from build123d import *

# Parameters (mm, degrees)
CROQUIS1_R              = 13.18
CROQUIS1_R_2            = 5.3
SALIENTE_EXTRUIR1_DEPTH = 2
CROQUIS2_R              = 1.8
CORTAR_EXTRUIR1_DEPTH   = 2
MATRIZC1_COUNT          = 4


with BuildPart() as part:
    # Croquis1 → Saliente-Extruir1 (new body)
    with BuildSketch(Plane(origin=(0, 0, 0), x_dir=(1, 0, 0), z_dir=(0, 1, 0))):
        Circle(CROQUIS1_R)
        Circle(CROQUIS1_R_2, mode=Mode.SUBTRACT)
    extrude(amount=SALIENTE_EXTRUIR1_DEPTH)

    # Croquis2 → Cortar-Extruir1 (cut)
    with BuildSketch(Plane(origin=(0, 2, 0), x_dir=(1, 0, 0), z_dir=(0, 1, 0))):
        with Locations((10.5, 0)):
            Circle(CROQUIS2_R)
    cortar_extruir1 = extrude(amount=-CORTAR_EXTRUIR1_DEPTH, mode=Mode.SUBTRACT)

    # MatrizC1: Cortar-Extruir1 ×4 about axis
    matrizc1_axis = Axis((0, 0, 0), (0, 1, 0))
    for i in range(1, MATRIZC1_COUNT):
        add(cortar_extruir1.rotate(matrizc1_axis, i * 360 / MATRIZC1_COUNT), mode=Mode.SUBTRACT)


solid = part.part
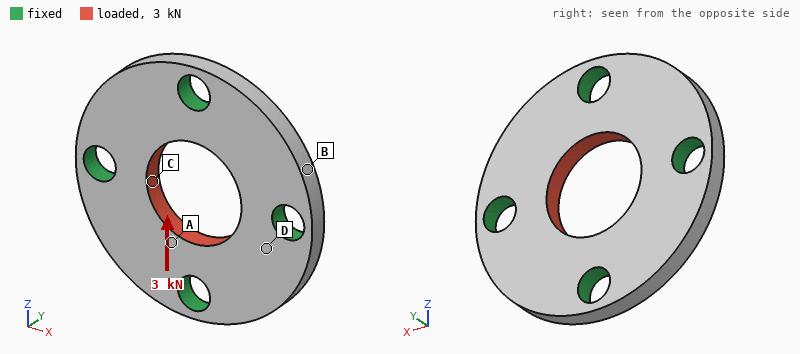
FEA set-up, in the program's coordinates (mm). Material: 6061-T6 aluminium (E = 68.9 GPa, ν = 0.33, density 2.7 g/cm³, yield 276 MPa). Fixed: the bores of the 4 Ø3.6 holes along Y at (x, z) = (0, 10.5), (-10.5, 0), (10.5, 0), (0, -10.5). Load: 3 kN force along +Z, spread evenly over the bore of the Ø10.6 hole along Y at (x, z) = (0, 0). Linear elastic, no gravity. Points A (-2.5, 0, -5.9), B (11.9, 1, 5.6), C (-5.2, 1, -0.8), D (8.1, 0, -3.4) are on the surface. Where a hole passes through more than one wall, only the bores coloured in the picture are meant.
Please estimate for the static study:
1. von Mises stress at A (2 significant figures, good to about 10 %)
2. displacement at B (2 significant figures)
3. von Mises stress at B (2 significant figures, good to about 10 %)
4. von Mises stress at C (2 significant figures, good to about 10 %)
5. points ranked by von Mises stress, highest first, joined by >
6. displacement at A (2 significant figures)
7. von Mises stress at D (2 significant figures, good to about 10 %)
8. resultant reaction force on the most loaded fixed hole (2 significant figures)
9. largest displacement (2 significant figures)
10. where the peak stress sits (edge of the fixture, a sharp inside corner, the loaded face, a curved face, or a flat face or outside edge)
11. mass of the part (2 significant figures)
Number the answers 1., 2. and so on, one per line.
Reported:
1. 63 MPa
2. 1.7 µm
3. 16 MPa
4. 78 MPa
5. C > A > D > B
6. 3.9 µm
7. 31 MPa
8. 860 N
9. 6.4 µm
10. edge of the fixture
11. 2.3 g
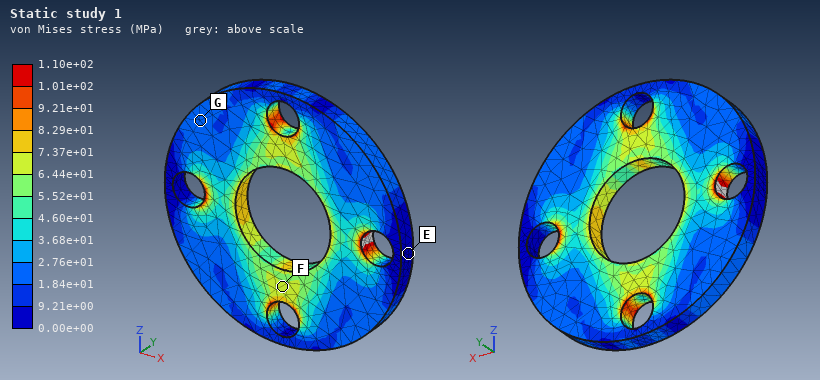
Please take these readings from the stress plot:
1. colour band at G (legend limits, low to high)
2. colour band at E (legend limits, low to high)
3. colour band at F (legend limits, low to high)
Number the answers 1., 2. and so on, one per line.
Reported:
1. 1.84e+01 to 2.76e+01 MPa
2. 0.00e+00 to 9.21e+00 MPa
3. 6.44e+01 to 7.37e+01 MPa
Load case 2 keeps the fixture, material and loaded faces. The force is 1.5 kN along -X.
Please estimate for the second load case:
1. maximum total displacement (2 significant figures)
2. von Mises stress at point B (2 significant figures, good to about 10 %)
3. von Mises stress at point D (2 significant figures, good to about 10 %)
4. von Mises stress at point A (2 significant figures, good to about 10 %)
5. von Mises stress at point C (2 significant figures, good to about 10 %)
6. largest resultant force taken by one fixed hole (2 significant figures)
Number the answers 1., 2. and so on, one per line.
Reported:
1. 3.2 µm
2. 9.1 MPa
3. 20 MPa
4. 20 MPa
5. 35 MPa
6. 430 N
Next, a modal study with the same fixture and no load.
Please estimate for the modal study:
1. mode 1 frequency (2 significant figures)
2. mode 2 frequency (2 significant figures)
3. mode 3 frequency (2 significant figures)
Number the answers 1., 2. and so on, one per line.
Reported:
1. 45 kHz
2. 45 kHz
3. 45 kHz
